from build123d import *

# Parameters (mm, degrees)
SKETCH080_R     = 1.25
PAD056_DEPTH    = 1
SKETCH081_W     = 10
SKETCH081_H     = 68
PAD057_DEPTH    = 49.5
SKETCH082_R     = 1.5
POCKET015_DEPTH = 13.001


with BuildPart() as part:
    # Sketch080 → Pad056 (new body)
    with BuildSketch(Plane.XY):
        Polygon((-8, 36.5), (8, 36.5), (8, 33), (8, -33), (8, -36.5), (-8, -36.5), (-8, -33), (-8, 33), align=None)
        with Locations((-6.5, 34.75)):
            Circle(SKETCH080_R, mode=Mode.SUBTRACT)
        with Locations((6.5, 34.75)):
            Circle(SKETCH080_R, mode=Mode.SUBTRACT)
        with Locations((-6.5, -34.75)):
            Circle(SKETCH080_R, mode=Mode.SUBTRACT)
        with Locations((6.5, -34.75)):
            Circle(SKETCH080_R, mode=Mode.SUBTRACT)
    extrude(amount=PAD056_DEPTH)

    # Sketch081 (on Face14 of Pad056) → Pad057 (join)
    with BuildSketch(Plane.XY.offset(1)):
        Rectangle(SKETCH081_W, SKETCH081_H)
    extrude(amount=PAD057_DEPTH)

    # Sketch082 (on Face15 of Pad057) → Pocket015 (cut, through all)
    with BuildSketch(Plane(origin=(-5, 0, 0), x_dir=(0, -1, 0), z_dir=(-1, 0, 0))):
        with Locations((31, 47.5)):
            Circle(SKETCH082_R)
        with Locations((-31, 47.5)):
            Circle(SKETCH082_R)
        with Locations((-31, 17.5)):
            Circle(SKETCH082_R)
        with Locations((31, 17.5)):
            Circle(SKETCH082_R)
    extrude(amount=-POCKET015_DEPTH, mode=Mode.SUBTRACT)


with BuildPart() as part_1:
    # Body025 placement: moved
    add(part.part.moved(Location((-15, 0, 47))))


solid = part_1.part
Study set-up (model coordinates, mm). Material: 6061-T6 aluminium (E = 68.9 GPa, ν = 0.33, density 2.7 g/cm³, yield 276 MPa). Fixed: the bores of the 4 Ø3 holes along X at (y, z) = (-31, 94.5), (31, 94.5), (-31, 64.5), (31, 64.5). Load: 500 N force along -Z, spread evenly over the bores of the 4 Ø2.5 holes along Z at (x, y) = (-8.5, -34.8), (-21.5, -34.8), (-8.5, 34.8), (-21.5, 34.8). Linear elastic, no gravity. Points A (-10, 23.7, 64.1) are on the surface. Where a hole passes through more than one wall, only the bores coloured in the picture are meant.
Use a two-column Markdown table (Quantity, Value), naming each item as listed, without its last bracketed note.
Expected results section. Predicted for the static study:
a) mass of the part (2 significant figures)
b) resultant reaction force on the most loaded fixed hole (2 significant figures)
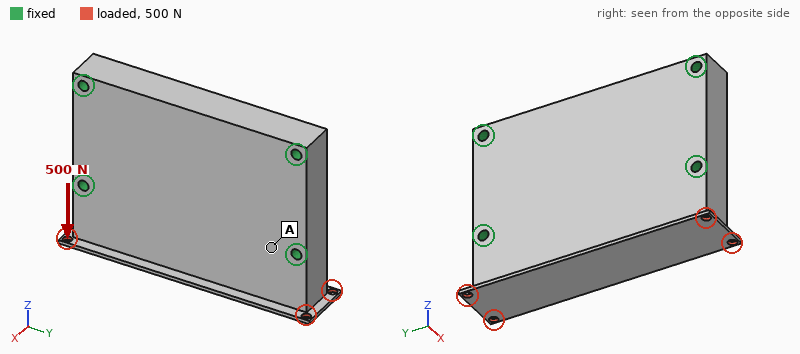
| Quantity | Value |
|---|---|
| mass of the part | 93 g |
| resultant reaction force on the most loaded fixed hole | 250 N |
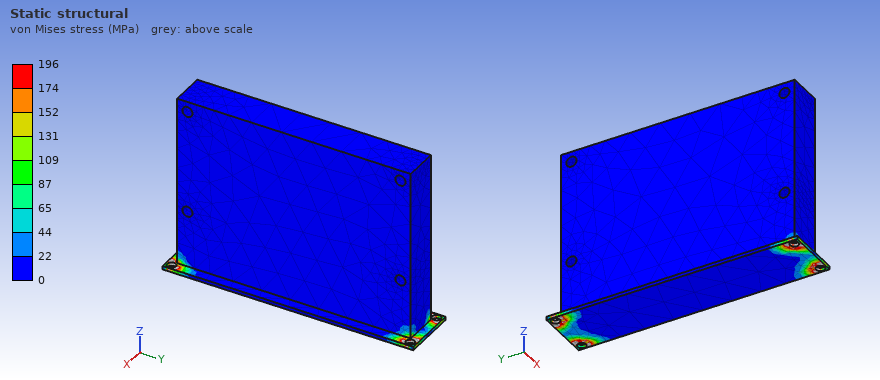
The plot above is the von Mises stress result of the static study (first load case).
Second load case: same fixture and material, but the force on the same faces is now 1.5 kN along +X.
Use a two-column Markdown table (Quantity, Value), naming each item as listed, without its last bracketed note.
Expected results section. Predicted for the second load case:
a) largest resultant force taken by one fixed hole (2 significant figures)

| Quantity | Value |
|---|---|
| largest resultant force taken by one fixed hole | 910 N |
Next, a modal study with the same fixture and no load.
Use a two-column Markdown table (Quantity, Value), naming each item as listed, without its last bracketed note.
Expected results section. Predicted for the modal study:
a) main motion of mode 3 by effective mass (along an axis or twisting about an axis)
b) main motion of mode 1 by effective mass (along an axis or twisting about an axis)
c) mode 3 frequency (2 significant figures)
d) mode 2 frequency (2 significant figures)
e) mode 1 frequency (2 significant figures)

| Quantity | Value |
|---|---|
| main motion of mode 3 by effective mass | twisting about Z |
| main motion of mode 1 by effective mass | along X |
| mode 3 frequency | 18 kHz |
| mode 2 frequency | 11 kHz |
| mode 1 frequency | 8600 Hz |
